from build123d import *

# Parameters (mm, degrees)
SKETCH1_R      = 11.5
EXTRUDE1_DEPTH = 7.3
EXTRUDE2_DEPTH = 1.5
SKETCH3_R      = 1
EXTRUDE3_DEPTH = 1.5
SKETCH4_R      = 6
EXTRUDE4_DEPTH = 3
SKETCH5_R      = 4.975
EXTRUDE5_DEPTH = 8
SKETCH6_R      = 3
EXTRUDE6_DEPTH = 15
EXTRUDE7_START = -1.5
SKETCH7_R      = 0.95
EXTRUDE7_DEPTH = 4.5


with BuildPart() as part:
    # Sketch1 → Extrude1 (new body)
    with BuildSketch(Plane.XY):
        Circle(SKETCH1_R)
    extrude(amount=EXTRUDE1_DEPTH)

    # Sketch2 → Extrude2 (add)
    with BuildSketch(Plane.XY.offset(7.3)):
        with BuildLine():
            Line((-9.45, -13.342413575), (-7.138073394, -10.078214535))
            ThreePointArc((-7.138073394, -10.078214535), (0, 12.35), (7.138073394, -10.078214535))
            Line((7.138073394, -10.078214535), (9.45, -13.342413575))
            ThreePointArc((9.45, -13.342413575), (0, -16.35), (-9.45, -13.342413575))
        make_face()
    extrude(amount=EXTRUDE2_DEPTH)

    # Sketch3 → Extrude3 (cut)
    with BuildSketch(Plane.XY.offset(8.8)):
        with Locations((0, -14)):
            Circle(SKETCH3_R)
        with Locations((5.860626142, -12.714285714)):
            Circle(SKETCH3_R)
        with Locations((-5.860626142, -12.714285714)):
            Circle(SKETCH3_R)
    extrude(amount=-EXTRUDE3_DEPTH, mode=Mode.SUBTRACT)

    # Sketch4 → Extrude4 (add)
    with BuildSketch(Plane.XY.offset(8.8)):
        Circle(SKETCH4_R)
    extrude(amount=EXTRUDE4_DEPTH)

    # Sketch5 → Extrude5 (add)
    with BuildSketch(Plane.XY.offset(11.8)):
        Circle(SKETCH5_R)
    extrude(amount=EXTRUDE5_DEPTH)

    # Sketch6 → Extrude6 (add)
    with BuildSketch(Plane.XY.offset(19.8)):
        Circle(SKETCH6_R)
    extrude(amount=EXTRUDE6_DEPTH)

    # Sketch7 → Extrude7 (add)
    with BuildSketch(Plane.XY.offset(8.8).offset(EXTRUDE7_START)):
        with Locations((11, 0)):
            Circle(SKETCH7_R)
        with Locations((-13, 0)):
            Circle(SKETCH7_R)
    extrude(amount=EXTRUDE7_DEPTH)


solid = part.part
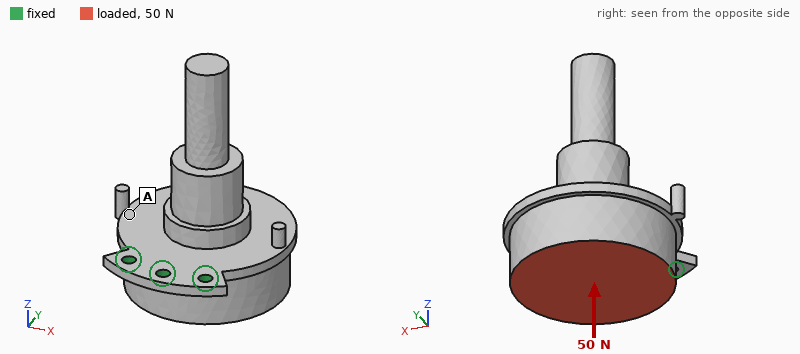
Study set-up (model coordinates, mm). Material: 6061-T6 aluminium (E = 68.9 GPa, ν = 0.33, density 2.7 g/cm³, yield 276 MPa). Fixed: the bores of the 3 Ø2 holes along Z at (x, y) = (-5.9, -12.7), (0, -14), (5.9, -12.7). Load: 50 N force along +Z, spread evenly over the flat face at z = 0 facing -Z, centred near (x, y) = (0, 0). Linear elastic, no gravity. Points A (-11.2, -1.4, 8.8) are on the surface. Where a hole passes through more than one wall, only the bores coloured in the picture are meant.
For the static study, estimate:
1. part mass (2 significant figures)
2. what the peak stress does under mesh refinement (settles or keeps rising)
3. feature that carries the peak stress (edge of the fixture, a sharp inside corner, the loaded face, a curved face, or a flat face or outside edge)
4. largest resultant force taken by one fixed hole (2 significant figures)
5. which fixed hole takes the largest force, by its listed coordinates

14 g
keeps rising
edge of the fixture
77 N
(0, -14)
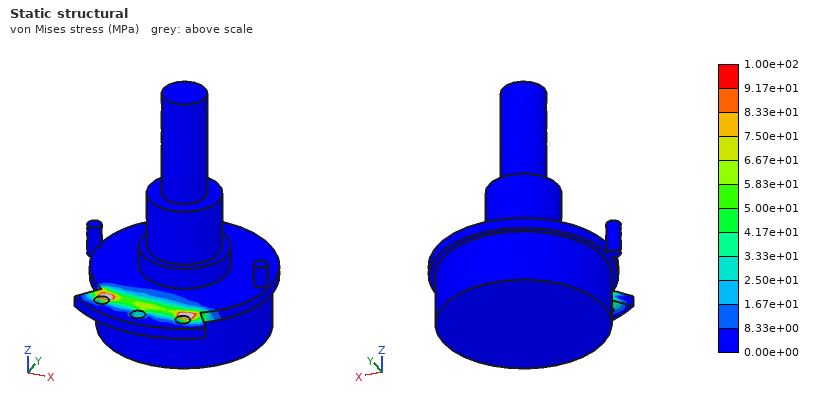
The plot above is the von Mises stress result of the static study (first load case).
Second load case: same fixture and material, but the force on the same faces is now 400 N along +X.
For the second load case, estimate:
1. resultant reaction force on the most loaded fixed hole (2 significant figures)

530 N
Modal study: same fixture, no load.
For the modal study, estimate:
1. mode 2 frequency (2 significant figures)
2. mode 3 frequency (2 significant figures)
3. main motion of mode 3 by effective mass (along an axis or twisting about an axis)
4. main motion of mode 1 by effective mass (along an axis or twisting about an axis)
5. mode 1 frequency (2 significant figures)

5000 Hz
7700 Hz
along X
along Z
1100 Hz
